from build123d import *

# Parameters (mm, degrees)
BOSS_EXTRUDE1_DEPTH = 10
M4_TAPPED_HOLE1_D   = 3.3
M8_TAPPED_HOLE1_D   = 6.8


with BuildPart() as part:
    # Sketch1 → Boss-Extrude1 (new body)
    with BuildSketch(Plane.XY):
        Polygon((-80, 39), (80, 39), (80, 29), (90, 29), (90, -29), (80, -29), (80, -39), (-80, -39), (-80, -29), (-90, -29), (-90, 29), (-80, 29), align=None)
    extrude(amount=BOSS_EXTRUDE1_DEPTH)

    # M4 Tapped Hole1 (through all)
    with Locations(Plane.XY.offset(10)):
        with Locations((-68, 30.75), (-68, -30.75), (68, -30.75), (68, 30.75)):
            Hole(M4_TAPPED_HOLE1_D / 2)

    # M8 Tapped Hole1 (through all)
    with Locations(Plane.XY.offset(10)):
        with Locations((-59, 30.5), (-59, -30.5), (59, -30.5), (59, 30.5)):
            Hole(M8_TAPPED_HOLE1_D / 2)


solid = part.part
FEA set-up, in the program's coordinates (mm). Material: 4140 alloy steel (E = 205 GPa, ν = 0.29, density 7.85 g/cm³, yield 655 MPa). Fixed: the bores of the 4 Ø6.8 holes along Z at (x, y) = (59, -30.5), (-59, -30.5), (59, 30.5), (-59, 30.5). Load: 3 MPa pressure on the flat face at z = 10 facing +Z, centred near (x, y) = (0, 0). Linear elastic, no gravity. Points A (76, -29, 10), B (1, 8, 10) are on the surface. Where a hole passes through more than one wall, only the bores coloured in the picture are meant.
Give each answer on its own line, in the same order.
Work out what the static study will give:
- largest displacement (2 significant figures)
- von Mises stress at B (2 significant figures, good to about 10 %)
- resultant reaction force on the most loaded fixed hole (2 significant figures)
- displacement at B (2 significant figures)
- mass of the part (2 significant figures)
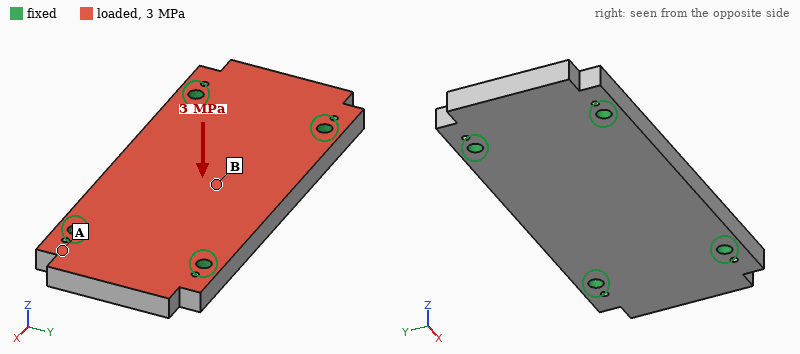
0.11 mm
94 MPa
10 kN
0.11 mm
1.1 kg
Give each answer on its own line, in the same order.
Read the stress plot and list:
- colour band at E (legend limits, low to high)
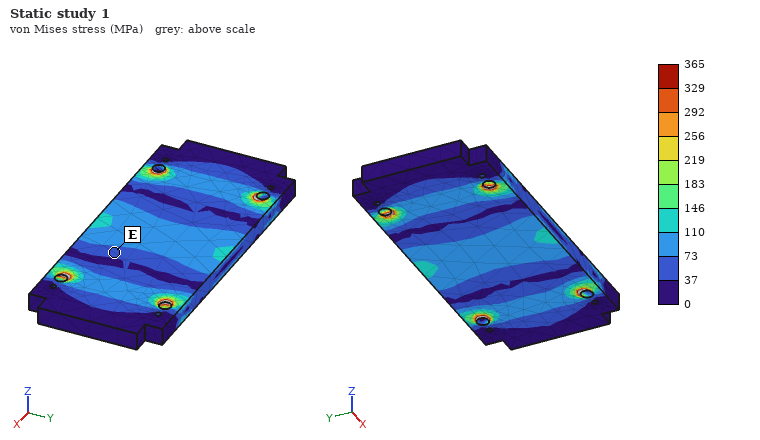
37 to 73 MPa
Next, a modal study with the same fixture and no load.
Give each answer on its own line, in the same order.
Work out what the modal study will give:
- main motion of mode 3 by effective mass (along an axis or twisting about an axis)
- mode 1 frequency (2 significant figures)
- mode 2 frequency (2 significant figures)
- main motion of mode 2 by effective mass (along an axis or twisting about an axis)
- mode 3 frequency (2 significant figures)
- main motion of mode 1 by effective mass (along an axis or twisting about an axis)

twisting about Y
3200 Hz
5100 Hz
twisting about X
6500 Hz
along Z
